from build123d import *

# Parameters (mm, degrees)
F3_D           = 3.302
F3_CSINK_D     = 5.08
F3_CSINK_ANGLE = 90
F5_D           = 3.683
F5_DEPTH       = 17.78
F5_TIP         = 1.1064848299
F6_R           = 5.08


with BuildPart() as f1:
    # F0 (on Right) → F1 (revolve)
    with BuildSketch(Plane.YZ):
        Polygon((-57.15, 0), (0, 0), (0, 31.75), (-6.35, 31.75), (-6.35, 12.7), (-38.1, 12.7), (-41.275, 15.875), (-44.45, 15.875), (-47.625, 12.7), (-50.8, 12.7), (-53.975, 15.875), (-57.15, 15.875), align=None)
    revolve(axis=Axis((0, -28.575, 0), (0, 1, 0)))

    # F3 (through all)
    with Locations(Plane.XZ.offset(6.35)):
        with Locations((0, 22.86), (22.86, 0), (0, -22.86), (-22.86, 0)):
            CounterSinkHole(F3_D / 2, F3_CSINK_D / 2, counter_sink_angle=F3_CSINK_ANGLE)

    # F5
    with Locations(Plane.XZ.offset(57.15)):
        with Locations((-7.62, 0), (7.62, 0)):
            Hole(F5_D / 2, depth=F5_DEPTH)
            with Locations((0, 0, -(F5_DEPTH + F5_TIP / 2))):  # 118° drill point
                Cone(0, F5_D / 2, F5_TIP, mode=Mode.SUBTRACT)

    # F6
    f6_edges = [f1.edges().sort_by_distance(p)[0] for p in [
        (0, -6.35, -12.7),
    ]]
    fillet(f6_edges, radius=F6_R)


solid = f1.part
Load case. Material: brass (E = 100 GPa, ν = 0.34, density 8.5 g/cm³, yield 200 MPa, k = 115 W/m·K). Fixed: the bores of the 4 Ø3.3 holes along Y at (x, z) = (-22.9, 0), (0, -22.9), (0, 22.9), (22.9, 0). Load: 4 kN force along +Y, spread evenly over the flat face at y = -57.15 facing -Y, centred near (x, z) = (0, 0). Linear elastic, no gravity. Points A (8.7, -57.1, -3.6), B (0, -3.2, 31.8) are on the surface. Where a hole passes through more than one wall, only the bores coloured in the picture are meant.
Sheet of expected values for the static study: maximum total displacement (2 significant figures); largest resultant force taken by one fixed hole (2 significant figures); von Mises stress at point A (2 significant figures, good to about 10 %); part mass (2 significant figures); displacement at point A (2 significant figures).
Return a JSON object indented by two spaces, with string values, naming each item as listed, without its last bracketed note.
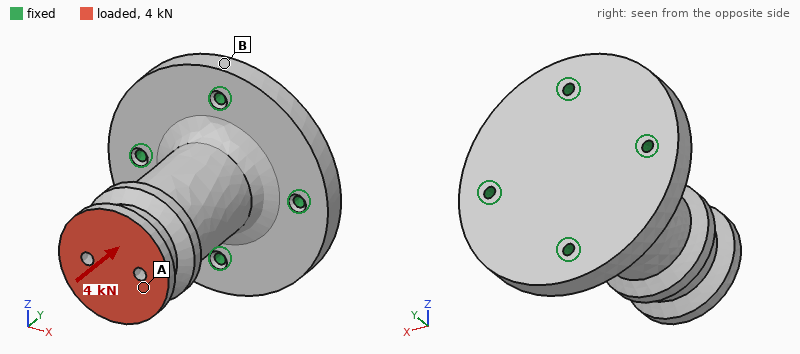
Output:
{
  "maximum total displacement": "11 µm",
  "largest resultant force taken by one fixed hole": "1.1 kN",
  "von Mises stress at point A": "10 MPa",
  "part mass": "420 g",
  "displacement at point A": "10 µm"
}
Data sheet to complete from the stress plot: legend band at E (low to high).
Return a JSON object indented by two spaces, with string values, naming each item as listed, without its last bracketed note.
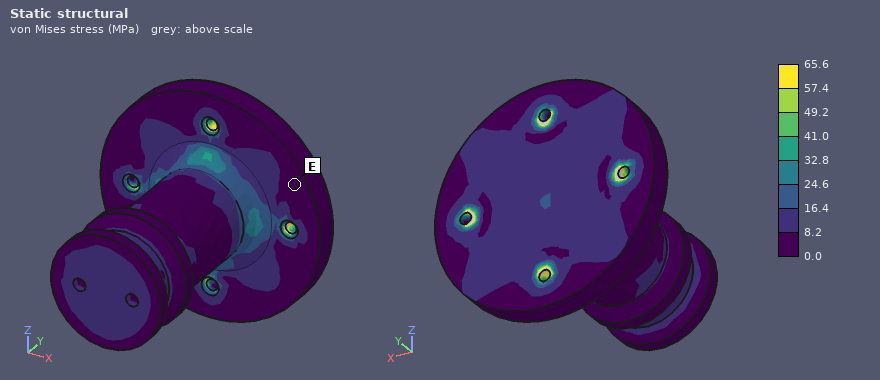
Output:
{
  "legend band at E": "0.0 to 8.2 MPa"
}
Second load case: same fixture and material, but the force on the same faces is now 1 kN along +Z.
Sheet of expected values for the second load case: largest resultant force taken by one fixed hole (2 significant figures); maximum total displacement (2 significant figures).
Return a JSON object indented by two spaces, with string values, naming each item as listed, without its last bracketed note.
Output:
{
  "largest resultant force taken by one fixed hole": "1.3 kN",
  "maximum total displacement": "48 µm"
}
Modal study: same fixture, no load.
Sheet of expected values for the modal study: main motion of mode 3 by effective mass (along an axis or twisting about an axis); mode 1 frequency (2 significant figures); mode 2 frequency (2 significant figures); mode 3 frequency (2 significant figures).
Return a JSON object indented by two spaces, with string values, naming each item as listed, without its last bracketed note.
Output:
{
  "main motion of mode 3 by effective mass": "along Y",
  "mode 1 frequency": "2600 Hz",
  "mode 2 frequency": "2600 Hz",
  "mode 3 frequency": "6700 Hz"
}
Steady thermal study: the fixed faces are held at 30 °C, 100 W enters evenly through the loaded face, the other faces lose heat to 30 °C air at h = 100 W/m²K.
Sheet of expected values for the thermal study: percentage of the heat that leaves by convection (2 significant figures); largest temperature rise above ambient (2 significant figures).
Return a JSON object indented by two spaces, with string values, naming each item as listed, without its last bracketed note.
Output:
{
  "percentage of the heat that leaves by convection": "32 %",
  "largest temperature rise above ambient": "85 K"
}
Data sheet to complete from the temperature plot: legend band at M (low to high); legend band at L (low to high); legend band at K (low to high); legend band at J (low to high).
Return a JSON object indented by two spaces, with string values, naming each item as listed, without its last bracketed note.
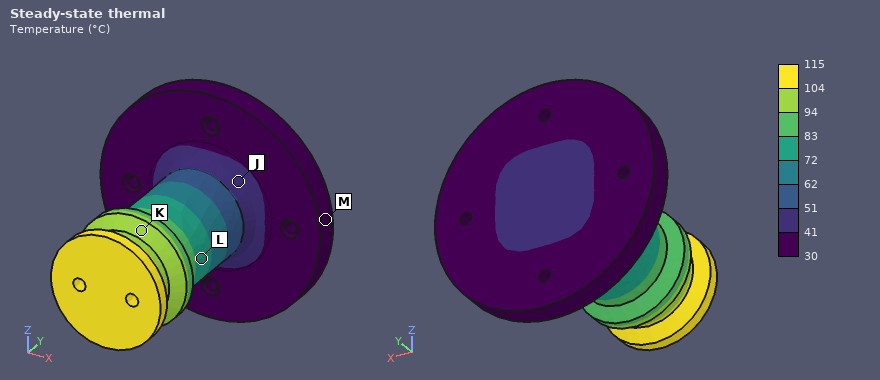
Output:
{
  "legend band at M": "30 to 41 °C",
  "legend band at L": "72 to 83 °C",
  "legend band at K": "94 to 104 °C",
  "legend band at J": "41 to 51 °C"
}
